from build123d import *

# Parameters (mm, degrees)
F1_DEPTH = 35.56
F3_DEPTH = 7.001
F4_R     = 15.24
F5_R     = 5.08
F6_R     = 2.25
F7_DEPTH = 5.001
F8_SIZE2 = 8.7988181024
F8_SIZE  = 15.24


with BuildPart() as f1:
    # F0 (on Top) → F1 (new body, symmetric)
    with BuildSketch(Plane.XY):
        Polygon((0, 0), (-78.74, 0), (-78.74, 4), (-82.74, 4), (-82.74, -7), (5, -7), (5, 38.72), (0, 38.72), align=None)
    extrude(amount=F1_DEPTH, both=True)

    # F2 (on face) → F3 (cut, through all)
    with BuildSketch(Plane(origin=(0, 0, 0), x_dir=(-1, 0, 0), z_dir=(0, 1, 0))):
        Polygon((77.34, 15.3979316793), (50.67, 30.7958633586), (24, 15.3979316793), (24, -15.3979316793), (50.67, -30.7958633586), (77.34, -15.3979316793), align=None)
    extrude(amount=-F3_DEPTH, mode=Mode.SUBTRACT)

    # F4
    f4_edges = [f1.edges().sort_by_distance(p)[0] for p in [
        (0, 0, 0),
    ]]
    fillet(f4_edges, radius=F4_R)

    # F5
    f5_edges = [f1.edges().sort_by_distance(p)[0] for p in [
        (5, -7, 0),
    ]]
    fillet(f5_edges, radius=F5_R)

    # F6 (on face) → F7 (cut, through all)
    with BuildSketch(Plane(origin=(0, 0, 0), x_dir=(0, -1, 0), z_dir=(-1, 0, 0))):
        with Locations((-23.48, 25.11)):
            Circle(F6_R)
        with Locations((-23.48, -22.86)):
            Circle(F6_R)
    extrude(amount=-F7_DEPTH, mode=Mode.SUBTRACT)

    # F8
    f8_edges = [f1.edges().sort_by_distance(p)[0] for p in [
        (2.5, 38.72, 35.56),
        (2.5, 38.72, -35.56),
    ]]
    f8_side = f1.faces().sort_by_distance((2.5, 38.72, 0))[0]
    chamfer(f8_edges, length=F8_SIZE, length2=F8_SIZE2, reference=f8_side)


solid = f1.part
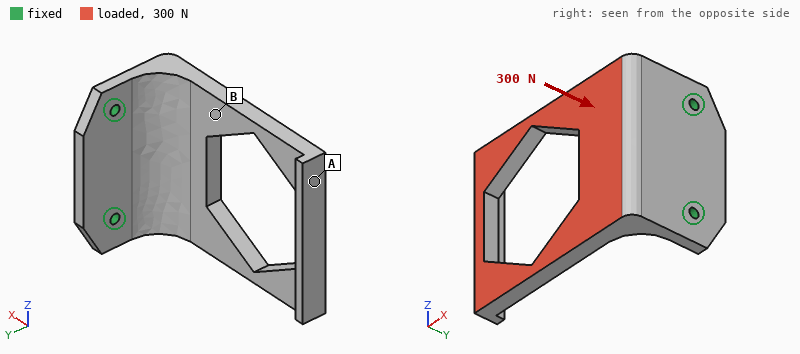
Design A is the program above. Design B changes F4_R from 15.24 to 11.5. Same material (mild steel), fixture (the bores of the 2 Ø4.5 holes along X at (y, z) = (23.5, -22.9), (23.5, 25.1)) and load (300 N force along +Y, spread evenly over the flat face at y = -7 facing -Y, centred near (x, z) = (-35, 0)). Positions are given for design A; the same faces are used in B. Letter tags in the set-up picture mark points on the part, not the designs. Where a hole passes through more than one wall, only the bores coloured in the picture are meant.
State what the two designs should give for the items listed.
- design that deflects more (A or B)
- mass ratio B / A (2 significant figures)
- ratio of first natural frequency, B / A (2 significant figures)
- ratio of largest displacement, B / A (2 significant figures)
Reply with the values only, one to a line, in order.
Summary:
B
0.97
0.95
1.1
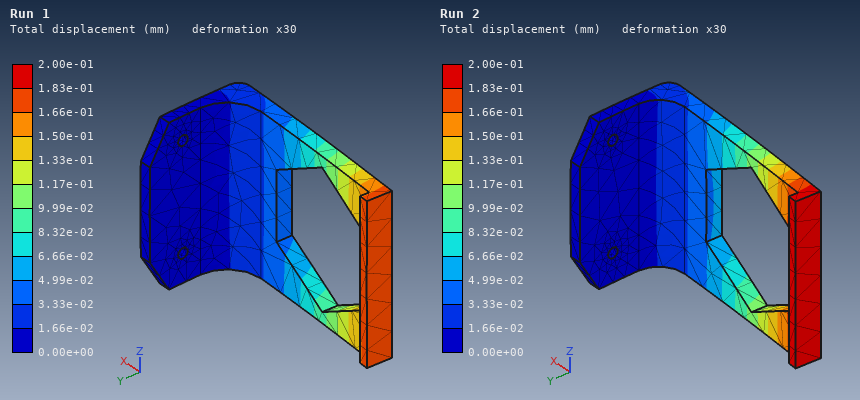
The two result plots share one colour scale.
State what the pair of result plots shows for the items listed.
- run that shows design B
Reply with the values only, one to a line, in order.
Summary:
Run 2
